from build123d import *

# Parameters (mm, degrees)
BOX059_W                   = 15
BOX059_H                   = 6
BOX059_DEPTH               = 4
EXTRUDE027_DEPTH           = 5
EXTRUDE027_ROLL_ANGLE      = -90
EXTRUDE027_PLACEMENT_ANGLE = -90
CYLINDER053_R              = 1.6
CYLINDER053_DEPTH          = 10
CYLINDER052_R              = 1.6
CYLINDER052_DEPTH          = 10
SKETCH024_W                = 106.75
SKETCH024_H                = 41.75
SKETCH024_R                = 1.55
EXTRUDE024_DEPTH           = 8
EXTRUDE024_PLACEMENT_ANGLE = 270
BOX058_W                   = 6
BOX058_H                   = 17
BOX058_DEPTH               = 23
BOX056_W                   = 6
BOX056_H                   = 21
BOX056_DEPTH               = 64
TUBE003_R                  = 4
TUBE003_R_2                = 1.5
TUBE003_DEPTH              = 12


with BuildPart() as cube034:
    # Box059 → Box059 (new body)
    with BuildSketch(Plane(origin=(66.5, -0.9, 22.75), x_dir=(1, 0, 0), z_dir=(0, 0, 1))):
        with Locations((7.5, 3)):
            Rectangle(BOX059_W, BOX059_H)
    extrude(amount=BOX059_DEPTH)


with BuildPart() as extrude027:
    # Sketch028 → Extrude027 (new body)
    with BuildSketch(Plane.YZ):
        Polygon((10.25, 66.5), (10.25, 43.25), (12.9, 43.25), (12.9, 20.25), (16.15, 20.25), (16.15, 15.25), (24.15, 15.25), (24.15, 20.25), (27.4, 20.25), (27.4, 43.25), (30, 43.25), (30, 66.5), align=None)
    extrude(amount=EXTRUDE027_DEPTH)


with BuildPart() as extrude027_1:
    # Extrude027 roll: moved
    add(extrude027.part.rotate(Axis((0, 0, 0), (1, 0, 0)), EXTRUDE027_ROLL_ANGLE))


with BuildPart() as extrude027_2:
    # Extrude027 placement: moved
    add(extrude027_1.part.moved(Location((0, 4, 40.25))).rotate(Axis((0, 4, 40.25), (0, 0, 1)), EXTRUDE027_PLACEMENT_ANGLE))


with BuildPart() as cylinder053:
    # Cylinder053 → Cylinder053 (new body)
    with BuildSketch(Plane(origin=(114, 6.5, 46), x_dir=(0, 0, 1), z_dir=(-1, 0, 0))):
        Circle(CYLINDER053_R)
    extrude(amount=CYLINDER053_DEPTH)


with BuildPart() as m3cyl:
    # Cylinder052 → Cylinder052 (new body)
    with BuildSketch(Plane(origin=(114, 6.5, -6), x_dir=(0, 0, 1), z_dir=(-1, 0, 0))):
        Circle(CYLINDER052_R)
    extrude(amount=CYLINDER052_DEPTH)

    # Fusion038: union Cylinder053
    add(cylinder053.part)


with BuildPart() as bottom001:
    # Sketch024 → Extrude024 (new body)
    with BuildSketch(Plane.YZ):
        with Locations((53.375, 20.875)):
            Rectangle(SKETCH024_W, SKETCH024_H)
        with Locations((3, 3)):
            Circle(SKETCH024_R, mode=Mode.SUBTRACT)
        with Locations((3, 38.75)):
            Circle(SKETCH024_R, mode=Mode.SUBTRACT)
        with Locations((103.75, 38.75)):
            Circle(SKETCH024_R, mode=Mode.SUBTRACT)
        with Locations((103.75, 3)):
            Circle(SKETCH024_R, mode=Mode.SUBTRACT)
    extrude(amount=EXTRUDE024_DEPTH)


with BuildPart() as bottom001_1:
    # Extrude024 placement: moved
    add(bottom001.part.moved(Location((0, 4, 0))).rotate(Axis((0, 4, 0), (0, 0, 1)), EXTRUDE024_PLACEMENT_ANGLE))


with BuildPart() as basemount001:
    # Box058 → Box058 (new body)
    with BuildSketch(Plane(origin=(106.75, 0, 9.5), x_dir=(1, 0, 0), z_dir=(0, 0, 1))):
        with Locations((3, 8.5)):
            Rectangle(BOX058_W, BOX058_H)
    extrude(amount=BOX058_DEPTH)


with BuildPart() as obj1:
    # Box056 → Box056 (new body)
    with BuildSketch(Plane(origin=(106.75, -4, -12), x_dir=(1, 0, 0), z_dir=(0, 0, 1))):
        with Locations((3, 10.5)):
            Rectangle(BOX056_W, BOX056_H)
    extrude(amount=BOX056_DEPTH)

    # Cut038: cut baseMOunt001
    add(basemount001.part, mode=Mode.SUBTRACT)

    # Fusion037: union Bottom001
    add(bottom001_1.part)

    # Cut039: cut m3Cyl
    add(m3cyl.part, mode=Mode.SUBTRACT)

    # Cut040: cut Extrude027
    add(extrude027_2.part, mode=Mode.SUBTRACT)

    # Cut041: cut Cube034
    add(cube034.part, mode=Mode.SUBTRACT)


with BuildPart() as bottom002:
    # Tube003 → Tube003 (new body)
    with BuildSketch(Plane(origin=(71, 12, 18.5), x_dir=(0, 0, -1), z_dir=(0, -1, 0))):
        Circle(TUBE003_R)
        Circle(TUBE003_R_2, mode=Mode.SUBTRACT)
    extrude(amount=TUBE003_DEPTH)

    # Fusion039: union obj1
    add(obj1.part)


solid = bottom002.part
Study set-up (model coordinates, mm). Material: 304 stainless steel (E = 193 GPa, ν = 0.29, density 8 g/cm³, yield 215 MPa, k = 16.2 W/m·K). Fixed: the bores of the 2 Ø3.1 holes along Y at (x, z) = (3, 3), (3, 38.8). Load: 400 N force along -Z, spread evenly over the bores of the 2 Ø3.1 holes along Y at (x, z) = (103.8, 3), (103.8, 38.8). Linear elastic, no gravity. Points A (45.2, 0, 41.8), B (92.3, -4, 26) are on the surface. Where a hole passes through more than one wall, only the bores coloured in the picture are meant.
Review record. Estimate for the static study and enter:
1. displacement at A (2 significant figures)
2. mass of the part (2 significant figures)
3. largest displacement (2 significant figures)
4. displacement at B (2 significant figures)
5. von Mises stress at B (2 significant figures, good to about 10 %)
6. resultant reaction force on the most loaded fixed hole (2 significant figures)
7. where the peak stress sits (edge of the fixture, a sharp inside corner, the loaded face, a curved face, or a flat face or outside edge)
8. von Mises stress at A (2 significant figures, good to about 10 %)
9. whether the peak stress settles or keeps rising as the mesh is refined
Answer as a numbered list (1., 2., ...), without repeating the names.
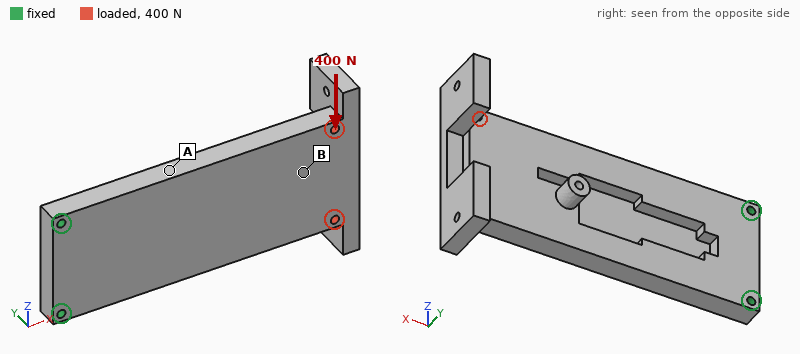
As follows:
1. 6.9 µm
2. 300 g
3. 29 µm
4. 16 µm
5. 3.0 MPa
6. 1.1 kN
7. edge of the fixture
8. 12 MPa
9. keeps rising
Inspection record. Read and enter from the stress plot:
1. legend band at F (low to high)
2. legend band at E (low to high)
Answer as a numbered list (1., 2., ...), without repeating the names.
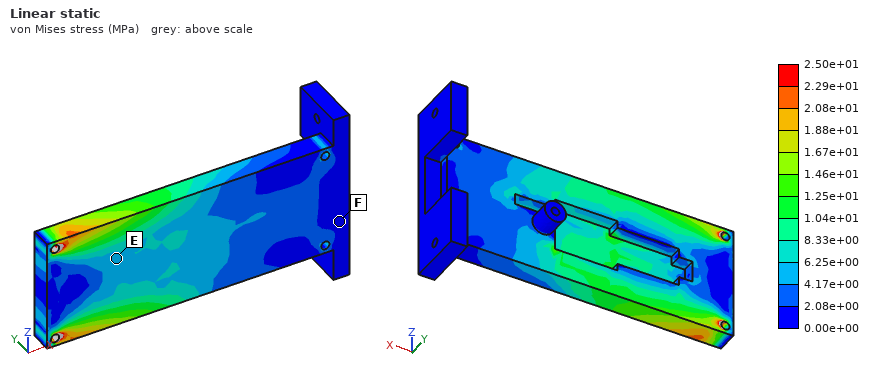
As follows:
1. 0.00e+00 to 2.08e+00 MPa
2. 4.17e+00 to 6.25e+00 MPa
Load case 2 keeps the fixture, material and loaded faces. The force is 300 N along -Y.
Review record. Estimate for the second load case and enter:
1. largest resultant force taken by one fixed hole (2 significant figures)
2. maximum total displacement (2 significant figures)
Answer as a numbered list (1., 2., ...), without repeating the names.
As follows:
1. 230 N
2. 0.50 mm
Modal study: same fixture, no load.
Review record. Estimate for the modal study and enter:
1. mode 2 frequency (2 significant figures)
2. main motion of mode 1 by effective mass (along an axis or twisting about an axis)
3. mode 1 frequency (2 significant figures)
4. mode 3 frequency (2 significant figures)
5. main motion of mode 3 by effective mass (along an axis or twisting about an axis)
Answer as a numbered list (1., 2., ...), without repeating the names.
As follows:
1. 1400 Hz
2. along Y
3. 380 Hz
4. 2100 Hz
5. along Z
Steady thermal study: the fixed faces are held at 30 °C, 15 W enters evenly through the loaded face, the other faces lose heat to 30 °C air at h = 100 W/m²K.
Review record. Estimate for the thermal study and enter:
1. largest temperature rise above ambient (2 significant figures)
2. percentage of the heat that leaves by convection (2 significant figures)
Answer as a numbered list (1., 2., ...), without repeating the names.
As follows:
1. 49 K
2. 99 %
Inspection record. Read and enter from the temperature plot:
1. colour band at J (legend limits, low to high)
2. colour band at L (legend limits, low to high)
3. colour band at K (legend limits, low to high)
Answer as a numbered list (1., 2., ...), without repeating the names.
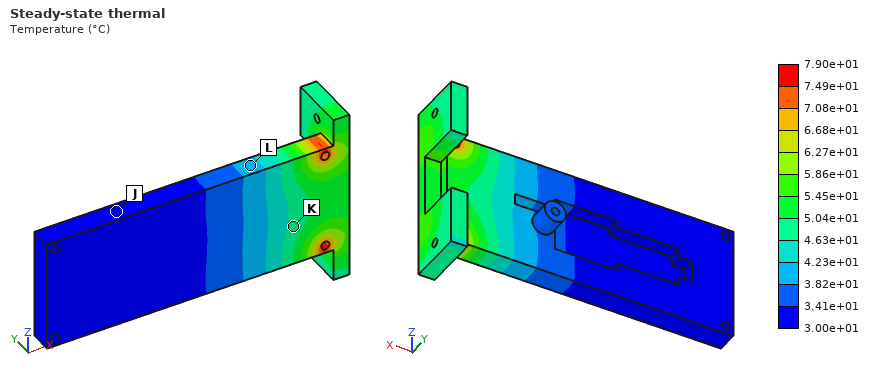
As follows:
1. 3.00e+01 to 3.41e+01 °C
2. 3.82e+01 to 4.23e+01 °C
3. 4.63e+01 to 5.04e+01 °C
